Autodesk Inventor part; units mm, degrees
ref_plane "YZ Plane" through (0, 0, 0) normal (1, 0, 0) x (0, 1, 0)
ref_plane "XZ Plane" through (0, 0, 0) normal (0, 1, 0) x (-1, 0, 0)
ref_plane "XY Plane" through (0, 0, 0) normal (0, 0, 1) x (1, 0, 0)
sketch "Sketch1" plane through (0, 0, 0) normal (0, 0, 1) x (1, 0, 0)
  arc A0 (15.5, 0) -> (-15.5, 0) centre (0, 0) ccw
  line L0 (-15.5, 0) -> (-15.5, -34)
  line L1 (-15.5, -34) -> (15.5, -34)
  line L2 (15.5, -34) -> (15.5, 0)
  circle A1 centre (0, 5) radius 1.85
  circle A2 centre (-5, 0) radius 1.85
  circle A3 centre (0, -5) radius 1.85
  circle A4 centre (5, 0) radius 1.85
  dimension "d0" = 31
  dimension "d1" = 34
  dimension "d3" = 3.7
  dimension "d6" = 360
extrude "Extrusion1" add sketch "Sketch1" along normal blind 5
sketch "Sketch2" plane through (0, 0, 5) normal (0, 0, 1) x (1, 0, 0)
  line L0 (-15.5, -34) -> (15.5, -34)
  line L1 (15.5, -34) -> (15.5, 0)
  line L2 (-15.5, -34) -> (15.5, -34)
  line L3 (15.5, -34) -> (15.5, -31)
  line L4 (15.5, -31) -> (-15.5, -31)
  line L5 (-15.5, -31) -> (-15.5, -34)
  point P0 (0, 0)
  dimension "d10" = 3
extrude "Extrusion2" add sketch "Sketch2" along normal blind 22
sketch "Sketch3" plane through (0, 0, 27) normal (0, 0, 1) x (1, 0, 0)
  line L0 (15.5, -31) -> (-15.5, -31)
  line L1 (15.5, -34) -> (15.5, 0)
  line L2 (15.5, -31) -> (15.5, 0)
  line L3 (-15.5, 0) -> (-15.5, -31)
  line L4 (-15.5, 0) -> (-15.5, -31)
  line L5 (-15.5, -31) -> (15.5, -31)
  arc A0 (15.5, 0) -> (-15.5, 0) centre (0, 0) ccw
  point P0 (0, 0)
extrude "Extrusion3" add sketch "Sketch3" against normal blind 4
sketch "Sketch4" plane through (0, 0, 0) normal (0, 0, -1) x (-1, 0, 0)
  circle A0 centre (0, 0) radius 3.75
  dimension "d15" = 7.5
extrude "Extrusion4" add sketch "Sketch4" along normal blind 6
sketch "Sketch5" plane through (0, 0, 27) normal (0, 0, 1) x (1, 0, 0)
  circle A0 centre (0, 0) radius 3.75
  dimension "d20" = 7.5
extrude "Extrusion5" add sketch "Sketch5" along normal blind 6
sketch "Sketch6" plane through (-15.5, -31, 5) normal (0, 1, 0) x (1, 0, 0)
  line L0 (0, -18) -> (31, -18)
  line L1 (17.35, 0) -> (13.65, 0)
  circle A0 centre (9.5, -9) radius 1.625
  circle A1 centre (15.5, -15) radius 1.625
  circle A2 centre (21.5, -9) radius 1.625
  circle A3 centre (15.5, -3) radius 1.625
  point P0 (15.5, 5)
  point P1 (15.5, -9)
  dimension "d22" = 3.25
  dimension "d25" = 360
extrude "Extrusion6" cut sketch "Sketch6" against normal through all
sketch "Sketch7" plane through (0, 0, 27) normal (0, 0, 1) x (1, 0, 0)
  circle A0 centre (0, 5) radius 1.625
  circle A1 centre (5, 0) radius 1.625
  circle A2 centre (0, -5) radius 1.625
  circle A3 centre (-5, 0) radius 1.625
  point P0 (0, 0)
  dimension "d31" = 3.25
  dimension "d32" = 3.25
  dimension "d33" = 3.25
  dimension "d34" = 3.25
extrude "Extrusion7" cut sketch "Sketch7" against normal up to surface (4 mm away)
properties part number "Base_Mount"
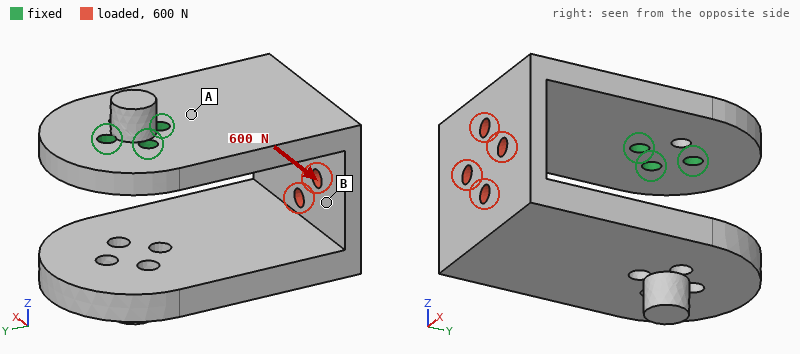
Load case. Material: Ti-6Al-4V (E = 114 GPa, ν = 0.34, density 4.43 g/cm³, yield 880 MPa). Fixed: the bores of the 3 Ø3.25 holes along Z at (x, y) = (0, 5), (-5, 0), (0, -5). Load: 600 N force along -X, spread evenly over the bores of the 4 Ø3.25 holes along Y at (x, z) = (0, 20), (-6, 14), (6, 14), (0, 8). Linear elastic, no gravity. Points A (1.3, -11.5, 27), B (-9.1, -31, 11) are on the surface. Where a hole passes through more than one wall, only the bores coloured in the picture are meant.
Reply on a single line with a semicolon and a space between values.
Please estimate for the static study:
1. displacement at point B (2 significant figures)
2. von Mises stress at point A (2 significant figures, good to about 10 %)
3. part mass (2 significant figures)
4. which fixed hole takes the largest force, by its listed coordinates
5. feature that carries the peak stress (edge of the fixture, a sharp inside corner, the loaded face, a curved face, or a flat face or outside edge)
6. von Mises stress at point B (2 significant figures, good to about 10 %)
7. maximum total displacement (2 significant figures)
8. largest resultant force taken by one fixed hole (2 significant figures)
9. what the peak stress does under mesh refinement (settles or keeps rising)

0.12 mm; 55 MPa; 65 g; (0, -5); edge of the fixture; 13 MPa; 0.24 mm; 1.5 kN; keeps rising
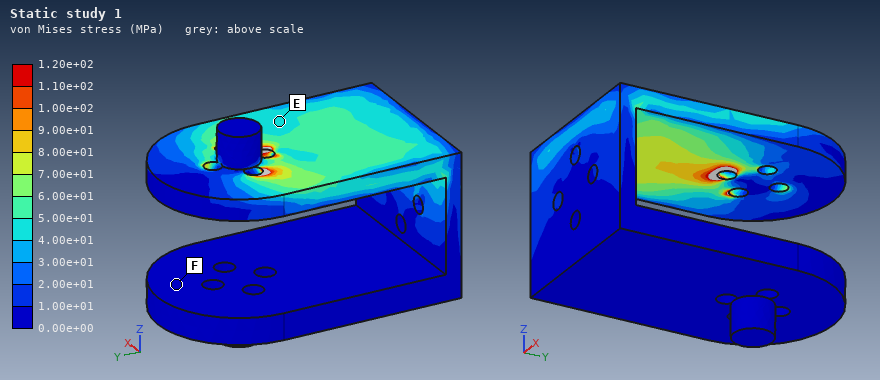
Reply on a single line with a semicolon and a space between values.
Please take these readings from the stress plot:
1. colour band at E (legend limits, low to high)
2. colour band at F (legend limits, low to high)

4.00e+01 to 5.00e+01 MPa; 0.00e+00 to 1.00e+01 MPa
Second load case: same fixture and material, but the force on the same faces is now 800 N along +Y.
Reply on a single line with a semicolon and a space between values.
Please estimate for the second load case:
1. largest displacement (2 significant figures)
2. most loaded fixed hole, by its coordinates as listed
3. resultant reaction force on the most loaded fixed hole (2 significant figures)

0.83 mm; (0, -5); 700 N
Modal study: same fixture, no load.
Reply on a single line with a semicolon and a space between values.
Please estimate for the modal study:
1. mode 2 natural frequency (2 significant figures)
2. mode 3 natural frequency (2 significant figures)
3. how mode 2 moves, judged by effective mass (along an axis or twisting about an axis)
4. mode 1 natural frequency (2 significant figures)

750 Hz; 1200 Hz; along X; 500 Hz
